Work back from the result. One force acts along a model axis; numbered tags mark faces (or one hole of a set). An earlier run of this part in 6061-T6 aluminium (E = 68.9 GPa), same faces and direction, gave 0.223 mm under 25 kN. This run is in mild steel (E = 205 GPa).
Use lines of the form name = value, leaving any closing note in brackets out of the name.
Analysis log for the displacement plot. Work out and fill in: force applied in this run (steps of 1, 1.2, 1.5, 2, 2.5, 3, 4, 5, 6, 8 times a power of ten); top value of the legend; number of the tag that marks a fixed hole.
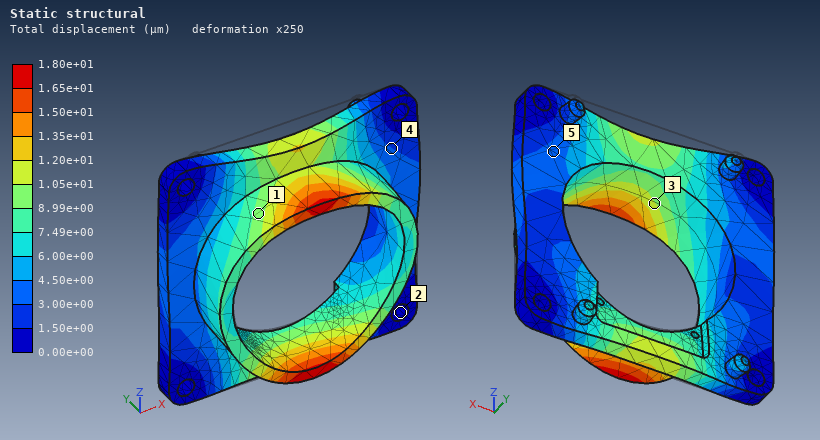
force applied in this run = 6 kN
top value of the legend = 1.80e+01 µm
number of the tag that marks a fixed hole = 2
